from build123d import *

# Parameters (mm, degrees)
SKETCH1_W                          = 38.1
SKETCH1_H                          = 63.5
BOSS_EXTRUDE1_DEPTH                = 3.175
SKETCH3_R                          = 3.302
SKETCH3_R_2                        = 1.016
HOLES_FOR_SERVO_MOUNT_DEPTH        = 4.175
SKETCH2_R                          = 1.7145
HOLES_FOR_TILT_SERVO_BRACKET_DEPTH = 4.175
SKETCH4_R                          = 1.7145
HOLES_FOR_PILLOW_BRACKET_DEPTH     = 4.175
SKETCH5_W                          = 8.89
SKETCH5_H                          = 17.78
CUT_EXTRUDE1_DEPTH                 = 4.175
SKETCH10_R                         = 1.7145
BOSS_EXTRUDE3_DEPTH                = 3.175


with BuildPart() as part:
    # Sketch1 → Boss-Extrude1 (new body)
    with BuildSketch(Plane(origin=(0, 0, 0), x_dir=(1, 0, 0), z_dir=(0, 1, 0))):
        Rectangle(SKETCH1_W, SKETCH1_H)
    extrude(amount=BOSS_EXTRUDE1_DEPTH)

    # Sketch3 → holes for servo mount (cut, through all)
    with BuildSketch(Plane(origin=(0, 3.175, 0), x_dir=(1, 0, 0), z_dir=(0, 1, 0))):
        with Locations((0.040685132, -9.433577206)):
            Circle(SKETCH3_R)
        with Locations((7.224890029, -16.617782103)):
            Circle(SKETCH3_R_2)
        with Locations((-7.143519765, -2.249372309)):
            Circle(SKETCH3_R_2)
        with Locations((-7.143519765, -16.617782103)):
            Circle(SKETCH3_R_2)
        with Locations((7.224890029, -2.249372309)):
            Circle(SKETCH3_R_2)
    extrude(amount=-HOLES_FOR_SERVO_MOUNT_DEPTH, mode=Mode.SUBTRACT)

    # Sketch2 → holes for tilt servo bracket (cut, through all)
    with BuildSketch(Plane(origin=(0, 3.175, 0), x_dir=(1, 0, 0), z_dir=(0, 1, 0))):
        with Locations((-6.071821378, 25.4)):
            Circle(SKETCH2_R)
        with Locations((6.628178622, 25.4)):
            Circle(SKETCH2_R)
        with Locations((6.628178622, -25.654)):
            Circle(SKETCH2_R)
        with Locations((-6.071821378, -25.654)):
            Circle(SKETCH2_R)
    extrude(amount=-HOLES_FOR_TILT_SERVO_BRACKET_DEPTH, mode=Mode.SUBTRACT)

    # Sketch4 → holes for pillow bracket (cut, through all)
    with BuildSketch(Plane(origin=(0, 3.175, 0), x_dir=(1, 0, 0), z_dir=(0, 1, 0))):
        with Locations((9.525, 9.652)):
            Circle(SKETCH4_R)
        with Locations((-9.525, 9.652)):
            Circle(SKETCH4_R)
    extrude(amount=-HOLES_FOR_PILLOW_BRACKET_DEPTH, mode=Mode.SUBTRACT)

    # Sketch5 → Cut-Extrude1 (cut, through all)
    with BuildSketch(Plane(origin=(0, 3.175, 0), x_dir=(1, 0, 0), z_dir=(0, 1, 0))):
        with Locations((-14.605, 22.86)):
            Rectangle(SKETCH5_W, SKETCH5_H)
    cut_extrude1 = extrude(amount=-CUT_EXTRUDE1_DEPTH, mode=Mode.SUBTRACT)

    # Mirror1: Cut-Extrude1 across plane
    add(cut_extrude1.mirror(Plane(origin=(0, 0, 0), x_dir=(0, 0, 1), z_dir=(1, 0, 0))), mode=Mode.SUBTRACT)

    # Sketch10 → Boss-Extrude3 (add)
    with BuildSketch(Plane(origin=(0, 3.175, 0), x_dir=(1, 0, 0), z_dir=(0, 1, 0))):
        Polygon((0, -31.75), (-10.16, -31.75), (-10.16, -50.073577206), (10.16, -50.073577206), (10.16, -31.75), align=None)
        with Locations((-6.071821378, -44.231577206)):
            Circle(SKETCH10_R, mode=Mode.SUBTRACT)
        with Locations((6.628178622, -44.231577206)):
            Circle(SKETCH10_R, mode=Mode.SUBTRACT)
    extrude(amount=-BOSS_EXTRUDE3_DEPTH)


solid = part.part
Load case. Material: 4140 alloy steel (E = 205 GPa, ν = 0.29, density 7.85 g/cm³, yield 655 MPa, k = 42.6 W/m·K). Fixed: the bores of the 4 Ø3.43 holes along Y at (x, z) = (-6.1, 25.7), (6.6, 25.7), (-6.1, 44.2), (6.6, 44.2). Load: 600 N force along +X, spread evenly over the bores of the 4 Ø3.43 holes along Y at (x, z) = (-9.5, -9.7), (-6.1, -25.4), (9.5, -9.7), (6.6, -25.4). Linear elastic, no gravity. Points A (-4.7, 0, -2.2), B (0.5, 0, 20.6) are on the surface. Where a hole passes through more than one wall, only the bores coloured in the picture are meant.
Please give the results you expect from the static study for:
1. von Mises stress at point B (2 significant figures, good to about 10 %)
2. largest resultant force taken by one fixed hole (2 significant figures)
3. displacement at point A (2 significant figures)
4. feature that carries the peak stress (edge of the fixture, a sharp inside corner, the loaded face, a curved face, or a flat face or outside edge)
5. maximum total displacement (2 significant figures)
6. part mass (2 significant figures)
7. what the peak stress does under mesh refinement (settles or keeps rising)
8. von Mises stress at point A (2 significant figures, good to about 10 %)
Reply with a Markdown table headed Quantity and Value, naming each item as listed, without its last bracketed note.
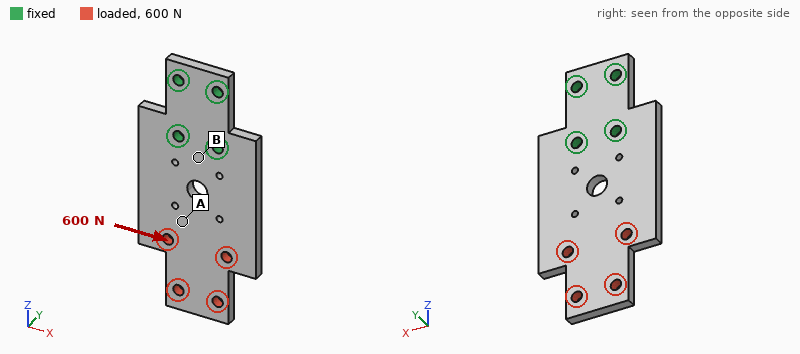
| Quantity | Value |
|---|---|
| von Mises stress at point B | 34 MPa |
| largest resultant force taken by one fixed hole | 1.4 kN |
| displacement at point A | 11 µm |
| feature that carries the peak stress | edge of the fixture |
| maximum total displacement | 26 µm |
| part mass | 59 g |
| what the peak stress does under mesh refinement | keeps rising |
| von Mises stress at point A | 13 MPa |
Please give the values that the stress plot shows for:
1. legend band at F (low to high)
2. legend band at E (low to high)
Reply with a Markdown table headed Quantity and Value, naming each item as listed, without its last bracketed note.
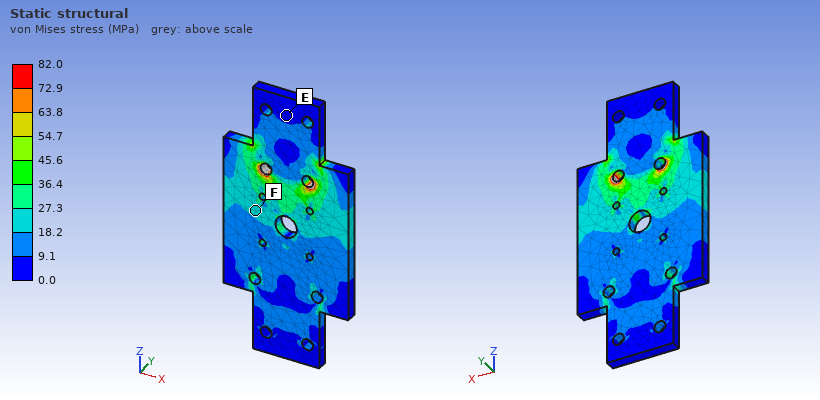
| Quantity | Value |
|---|---|
| legend band at F | 18.2 to 27.3 MPa |
| legend band at E | 0.0 to 9.1 MPa |
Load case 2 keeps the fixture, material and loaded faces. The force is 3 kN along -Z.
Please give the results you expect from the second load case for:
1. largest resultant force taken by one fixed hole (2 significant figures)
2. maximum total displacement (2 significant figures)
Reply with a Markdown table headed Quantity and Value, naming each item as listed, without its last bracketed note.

| Quantity | Value |
|---|---|
| largest resultant force taken by one fixed hole | 1.4 kN |
| maximum total displacement | 9.3 µm |
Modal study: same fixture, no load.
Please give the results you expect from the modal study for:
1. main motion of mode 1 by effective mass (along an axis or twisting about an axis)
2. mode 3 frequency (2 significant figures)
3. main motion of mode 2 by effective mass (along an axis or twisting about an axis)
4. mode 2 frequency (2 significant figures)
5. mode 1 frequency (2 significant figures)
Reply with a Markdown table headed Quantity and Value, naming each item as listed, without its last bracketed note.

| Quantity | Value |
|---|---|
| main motion of mode 1 by effective mass | along Y |
| mode 3 frequency | 4700 Hz |
| main motion of mode 2 by effective mass | twisting about Z |
| mode 2 frequency | 3400 Hz |
| mode 1 frequency | 980 Hz |
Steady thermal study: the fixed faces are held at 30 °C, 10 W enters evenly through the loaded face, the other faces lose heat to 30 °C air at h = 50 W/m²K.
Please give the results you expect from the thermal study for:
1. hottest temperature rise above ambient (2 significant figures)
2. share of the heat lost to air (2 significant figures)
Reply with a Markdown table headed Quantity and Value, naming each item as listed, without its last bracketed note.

| Quantity | Value |
|---|---|
| hottest temperature rise above ambient | 62 K |
| share of the heat lost to air | 59 % |
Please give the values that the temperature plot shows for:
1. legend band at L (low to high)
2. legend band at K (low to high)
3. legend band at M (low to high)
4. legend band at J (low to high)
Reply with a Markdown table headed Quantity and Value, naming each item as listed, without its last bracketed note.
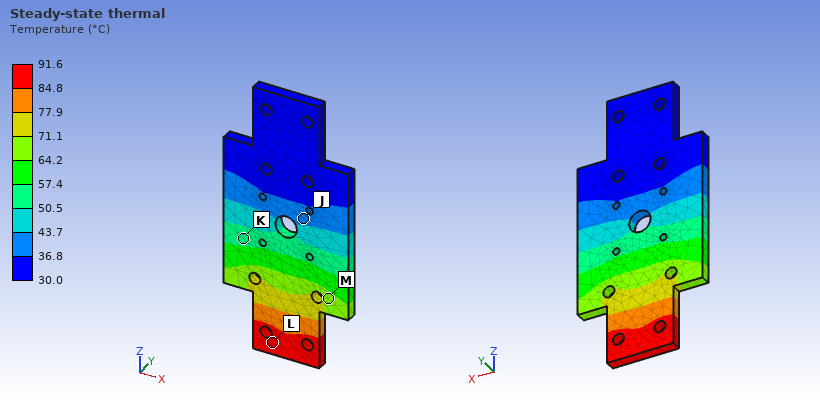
| Quantity | Value |
|---|---|
| legend band at L | 84.8 to 91.6 °C |
| legend band at K | 50.5 to 57.4 °C |
| legend band at M | 64.2 to 71.1 °C |
| legend band at J | 36.8 to 43.7 °C |
